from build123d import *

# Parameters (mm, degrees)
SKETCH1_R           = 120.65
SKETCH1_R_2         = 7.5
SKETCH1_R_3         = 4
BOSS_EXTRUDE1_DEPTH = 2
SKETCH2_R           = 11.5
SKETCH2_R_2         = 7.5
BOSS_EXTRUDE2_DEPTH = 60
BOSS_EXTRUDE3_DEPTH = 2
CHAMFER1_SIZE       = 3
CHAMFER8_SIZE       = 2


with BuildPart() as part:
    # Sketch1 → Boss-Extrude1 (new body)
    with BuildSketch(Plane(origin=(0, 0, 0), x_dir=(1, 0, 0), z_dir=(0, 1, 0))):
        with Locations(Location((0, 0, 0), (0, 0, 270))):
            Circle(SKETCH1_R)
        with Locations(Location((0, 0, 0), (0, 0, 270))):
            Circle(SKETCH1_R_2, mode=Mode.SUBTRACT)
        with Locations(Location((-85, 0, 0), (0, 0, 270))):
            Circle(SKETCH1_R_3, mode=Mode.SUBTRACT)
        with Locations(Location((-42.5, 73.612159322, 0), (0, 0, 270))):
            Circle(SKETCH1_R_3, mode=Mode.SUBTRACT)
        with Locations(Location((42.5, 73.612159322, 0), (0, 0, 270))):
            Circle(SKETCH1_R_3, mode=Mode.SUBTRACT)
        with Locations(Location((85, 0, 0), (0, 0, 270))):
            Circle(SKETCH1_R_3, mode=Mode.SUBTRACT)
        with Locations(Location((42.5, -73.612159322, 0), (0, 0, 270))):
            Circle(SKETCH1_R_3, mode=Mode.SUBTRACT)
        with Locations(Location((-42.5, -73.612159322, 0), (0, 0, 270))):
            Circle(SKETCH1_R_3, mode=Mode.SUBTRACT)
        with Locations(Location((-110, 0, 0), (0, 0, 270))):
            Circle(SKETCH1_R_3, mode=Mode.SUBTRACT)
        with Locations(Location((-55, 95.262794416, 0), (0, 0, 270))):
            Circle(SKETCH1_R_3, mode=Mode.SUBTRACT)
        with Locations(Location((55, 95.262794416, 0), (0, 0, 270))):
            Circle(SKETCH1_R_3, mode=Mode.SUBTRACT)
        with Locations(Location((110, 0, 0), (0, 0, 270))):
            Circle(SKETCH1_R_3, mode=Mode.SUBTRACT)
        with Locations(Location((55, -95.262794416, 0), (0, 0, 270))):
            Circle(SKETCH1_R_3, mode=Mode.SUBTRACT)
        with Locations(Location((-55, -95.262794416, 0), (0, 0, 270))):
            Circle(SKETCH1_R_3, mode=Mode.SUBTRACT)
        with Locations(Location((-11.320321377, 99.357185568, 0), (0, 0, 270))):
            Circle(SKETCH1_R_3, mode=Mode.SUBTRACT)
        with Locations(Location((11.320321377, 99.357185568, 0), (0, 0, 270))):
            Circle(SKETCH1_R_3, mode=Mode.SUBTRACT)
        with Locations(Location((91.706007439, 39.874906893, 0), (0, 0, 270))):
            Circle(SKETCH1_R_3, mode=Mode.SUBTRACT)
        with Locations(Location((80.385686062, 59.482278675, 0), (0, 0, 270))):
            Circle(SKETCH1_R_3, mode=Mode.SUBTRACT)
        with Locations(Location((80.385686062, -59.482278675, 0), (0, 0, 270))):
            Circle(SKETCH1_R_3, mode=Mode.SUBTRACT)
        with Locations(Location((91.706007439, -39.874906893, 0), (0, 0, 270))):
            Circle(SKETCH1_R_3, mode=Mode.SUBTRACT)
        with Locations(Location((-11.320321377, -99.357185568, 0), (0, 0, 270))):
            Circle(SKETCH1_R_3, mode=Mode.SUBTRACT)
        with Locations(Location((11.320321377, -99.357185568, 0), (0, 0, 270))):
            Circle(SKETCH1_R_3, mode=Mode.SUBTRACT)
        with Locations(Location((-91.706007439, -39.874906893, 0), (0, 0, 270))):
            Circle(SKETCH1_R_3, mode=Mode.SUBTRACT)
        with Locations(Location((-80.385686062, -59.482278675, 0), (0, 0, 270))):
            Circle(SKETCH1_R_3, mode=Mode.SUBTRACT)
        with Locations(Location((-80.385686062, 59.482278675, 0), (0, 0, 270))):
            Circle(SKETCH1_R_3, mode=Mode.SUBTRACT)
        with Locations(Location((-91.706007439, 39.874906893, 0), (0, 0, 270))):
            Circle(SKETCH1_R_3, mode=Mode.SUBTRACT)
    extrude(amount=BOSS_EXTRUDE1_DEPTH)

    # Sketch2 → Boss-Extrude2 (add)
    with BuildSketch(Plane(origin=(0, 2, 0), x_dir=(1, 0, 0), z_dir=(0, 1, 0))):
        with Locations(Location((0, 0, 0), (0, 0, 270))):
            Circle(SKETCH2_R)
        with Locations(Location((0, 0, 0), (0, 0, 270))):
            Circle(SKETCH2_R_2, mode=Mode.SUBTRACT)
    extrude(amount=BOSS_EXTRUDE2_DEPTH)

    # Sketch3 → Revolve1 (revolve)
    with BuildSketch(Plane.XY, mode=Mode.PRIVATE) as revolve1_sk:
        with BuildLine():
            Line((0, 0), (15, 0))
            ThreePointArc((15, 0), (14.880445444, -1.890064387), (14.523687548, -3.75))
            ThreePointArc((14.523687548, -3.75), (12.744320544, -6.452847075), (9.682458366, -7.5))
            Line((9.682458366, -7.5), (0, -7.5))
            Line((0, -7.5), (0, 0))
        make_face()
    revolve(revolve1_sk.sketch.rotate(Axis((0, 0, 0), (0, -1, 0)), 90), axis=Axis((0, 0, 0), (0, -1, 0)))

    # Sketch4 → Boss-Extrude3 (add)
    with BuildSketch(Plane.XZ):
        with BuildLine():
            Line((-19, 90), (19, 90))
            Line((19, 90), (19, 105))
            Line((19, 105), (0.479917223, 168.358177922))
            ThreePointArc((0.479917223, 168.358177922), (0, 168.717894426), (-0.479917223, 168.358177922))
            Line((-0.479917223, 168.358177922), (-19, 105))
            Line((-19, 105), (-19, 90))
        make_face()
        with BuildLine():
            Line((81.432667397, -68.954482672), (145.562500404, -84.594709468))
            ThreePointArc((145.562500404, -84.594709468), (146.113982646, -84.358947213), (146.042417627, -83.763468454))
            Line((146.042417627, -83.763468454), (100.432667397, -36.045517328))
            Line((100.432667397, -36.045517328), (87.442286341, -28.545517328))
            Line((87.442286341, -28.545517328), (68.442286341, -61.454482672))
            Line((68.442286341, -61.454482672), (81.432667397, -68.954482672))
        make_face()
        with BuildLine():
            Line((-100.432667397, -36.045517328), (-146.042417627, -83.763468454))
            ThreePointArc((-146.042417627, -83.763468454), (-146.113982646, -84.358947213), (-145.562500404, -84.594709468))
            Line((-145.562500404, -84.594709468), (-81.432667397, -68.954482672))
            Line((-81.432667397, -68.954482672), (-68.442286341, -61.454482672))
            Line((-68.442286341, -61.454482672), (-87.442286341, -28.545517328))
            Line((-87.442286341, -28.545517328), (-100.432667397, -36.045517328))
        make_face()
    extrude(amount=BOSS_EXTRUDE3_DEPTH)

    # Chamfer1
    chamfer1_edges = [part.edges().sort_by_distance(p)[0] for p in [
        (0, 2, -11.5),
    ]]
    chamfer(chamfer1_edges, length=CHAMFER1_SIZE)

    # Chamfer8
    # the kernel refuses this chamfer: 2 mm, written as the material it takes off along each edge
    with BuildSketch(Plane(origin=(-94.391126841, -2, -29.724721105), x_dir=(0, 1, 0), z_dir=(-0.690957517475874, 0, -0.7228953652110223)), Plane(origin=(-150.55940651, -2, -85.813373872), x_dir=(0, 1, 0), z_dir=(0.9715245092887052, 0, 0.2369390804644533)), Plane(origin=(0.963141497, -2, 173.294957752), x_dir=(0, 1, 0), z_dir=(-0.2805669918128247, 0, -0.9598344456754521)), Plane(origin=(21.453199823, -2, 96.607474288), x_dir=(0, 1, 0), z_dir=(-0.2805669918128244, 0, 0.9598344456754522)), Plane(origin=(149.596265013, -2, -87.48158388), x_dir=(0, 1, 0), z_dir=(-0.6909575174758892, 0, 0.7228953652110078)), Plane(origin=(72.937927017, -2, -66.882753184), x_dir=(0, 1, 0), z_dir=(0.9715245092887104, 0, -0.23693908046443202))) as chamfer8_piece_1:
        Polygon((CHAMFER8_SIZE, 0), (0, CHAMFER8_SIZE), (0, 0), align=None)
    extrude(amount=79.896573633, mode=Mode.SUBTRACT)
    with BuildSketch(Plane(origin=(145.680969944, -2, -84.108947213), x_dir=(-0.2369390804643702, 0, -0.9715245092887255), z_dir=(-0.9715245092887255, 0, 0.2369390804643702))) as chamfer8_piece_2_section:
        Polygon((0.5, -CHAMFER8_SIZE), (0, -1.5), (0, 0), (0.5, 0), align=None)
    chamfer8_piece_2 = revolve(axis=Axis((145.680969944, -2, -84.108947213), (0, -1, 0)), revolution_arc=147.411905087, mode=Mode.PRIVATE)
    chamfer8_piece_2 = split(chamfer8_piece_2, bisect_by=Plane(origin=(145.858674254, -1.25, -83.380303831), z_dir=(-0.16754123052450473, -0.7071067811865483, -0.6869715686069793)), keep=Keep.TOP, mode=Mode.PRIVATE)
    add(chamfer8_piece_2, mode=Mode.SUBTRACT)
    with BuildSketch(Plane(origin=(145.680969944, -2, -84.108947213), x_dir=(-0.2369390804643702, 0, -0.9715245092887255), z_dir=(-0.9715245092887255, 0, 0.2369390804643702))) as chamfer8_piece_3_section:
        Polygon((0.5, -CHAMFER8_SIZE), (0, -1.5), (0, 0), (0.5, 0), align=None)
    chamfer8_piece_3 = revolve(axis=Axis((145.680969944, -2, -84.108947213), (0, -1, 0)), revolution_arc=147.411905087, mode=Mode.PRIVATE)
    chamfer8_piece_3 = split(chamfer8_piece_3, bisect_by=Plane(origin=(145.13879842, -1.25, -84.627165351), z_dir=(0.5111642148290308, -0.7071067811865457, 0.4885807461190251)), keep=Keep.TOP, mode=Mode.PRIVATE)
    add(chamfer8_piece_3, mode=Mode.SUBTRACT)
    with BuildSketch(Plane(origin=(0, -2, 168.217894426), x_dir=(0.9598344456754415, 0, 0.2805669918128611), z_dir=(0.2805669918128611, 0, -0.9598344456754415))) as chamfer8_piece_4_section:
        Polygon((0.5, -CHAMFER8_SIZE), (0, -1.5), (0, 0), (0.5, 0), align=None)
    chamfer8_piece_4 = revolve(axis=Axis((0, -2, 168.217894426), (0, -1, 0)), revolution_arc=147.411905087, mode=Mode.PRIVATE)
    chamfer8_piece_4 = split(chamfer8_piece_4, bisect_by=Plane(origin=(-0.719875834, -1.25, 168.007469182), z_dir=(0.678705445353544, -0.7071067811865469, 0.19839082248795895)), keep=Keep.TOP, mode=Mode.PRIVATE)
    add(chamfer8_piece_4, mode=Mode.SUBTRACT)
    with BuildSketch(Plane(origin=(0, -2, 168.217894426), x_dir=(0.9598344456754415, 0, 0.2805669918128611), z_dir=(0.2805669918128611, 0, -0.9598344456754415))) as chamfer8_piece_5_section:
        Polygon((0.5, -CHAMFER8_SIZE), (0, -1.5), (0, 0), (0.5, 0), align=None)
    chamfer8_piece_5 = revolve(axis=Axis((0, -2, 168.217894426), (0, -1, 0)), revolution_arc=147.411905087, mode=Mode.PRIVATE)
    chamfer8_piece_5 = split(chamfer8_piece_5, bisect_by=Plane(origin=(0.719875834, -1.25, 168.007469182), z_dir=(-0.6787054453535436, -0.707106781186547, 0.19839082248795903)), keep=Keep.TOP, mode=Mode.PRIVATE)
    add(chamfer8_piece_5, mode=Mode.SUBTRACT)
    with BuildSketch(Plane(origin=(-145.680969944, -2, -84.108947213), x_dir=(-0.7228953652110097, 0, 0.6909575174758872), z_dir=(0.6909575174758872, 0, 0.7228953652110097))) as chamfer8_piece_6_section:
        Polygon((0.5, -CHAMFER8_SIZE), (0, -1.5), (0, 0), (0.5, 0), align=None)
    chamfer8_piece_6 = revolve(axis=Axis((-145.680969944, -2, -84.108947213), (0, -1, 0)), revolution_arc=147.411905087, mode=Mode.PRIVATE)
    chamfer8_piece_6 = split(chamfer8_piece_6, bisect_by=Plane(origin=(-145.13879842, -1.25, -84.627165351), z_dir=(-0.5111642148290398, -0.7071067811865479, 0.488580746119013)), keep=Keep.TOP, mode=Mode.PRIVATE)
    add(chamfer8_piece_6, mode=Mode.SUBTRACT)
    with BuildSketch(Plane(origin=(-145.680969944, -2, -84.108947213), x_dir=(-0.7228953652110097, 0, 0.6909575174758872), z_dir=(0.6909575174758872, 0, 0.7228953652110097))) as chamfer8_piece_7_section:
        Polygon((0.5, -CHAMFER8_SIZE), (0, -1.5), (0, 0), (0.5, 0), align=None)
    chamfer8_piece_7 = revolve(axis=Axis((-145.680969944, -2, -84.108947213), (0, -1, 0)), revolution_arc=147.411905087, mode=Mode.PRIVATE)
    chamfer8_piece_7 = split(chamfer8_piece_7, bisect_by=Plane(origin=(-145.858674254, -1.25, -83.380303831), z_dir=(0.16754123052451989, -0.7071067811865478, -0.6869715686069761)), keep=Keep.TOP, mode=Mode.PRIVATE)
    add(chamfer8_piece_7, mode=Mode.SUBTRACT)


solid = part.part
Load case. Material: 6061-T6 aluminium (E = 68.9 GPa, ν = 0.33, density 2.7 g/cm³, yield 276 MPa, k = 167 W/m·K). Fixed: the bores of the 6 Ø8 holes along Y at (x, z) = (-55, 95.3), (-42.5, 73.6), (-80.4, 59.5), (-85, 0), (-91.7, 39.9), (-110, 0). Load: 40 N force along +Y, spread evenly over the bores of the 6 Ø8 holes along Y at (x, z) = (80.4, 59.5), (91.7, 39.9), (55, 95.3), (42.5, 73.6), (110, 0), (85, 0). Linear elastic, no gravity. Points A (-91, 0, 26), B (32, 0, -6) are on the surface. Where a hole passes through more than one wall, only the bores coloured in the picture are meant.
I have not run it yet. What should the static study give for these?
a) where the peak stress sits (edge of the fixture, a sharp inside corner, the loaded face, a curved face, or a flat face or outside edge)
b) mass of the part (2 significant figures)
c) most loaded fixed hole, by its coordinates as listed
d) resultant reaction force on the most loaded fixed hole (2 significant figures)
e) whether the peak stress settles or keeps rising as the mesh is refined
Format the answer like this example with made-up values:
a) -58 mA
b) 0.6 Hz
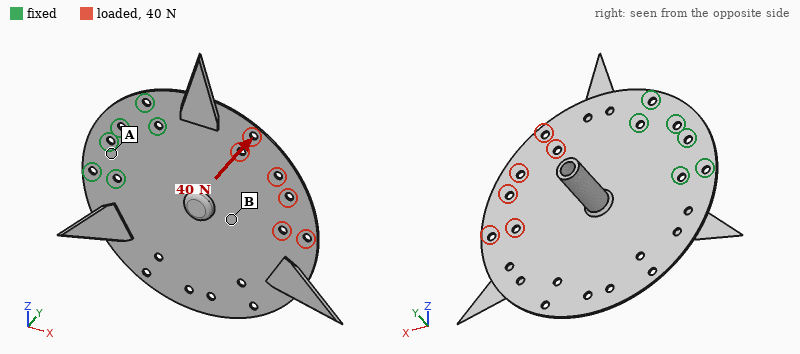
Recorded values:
a) edge of the fixture
b) 320 g
c) (-42.5, 73.6)
d) 110 N
e) keeps rising
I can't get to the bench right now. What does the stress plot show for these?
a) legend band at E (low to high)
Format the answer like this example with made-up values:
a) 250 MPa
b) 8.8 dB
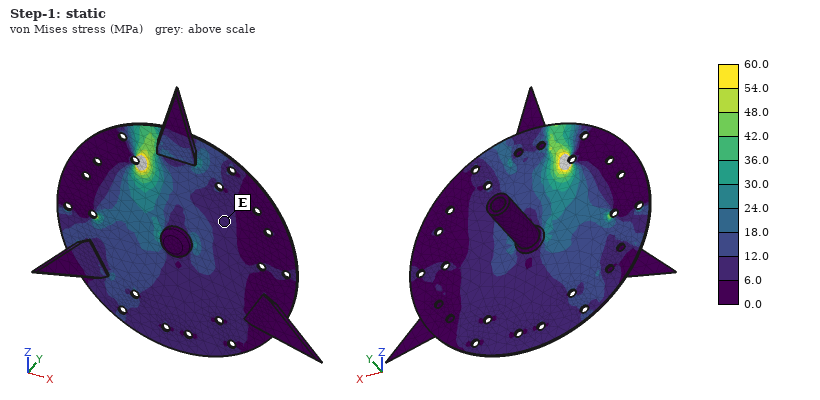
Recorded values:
a) 6.0 to 12.0 MPa
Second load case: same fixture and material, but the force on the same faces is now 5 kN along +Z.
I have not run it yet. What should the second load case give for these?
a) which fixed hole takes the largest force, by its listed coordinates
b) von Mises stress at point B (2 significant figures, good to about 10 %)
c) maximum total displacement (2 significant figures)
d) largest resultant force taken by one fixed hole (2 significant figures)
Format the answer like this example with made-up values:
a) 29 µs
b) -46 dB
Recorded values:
a) (-42.5, 73.6)
b) 23 MPa
c) 0.39 mm
d) 5.2 kN
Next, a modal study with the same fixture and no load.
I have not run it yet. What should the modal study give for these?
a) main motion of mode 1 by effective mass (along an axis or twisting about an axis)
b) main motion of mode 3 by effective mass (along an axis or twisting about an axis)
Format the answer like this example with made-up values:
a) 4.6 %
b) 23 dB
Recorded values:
a) along Y
b) along Y
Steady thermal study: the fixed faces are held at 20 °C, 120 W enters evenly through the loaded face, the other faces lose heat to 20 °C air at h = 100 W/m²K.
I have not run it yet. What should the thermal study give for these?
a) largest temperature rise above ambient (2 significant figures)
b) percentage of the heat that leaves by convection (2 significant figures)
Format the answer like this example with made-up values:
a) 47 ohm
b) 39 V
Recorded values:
a) 66 K
b) 96 %
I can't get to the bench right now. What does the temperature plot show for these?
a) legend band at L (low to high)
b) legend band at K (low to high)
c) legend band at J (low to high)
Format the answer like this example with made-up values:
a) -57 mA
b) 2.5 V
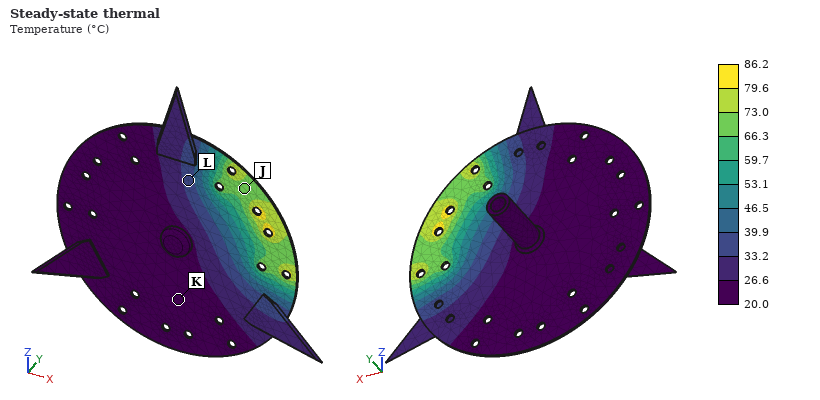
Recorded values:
a) 33.2 to 39.9 °C
b) 20.0 to 26.6 °C
c) 66.3 to 73.0 °C
